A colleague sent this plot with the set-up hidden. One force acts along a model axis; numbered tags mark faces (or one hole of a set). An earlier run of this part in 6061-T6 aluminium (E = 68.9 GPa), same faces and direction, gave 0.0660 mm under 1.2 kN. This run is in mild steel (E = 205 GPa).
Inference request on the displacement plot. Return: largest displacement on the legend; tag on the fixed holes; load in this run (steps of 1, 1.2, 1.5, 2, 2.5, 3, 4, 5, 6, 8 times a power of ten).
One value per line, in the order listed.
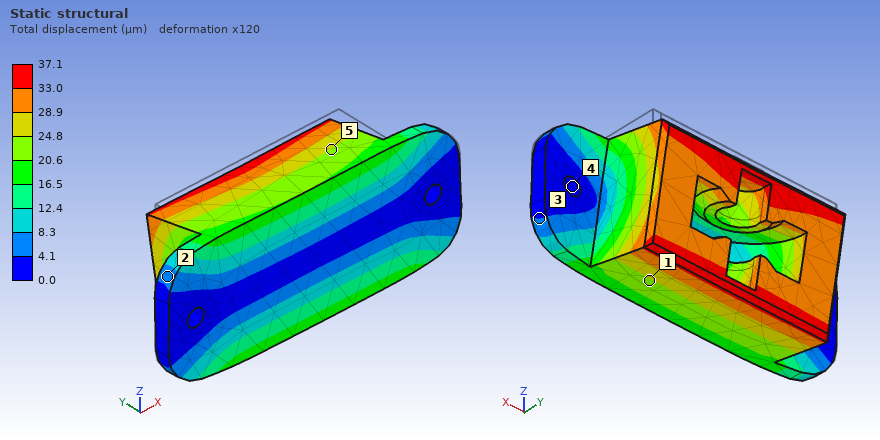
37.1 µm
4
2 kN
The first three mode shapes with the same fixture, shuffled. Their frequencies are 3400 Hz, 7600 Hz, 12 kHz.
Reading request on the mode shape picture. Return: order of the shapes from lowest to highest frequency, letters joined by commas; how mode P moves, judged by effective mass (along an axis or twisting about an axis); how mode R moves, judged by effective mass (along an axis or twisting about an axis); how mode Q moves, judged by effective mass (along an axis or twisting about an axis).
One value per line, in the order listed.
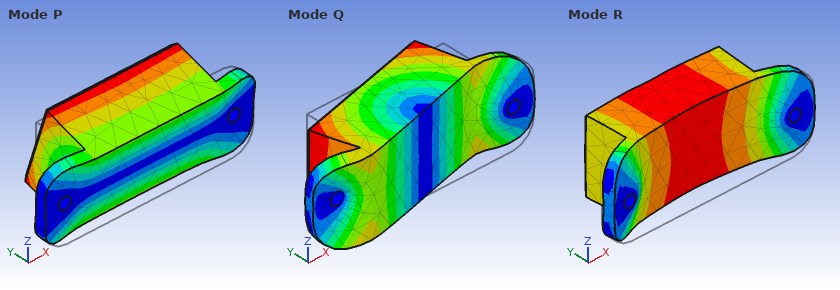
P, R, Q
along Z
along Y
along X
